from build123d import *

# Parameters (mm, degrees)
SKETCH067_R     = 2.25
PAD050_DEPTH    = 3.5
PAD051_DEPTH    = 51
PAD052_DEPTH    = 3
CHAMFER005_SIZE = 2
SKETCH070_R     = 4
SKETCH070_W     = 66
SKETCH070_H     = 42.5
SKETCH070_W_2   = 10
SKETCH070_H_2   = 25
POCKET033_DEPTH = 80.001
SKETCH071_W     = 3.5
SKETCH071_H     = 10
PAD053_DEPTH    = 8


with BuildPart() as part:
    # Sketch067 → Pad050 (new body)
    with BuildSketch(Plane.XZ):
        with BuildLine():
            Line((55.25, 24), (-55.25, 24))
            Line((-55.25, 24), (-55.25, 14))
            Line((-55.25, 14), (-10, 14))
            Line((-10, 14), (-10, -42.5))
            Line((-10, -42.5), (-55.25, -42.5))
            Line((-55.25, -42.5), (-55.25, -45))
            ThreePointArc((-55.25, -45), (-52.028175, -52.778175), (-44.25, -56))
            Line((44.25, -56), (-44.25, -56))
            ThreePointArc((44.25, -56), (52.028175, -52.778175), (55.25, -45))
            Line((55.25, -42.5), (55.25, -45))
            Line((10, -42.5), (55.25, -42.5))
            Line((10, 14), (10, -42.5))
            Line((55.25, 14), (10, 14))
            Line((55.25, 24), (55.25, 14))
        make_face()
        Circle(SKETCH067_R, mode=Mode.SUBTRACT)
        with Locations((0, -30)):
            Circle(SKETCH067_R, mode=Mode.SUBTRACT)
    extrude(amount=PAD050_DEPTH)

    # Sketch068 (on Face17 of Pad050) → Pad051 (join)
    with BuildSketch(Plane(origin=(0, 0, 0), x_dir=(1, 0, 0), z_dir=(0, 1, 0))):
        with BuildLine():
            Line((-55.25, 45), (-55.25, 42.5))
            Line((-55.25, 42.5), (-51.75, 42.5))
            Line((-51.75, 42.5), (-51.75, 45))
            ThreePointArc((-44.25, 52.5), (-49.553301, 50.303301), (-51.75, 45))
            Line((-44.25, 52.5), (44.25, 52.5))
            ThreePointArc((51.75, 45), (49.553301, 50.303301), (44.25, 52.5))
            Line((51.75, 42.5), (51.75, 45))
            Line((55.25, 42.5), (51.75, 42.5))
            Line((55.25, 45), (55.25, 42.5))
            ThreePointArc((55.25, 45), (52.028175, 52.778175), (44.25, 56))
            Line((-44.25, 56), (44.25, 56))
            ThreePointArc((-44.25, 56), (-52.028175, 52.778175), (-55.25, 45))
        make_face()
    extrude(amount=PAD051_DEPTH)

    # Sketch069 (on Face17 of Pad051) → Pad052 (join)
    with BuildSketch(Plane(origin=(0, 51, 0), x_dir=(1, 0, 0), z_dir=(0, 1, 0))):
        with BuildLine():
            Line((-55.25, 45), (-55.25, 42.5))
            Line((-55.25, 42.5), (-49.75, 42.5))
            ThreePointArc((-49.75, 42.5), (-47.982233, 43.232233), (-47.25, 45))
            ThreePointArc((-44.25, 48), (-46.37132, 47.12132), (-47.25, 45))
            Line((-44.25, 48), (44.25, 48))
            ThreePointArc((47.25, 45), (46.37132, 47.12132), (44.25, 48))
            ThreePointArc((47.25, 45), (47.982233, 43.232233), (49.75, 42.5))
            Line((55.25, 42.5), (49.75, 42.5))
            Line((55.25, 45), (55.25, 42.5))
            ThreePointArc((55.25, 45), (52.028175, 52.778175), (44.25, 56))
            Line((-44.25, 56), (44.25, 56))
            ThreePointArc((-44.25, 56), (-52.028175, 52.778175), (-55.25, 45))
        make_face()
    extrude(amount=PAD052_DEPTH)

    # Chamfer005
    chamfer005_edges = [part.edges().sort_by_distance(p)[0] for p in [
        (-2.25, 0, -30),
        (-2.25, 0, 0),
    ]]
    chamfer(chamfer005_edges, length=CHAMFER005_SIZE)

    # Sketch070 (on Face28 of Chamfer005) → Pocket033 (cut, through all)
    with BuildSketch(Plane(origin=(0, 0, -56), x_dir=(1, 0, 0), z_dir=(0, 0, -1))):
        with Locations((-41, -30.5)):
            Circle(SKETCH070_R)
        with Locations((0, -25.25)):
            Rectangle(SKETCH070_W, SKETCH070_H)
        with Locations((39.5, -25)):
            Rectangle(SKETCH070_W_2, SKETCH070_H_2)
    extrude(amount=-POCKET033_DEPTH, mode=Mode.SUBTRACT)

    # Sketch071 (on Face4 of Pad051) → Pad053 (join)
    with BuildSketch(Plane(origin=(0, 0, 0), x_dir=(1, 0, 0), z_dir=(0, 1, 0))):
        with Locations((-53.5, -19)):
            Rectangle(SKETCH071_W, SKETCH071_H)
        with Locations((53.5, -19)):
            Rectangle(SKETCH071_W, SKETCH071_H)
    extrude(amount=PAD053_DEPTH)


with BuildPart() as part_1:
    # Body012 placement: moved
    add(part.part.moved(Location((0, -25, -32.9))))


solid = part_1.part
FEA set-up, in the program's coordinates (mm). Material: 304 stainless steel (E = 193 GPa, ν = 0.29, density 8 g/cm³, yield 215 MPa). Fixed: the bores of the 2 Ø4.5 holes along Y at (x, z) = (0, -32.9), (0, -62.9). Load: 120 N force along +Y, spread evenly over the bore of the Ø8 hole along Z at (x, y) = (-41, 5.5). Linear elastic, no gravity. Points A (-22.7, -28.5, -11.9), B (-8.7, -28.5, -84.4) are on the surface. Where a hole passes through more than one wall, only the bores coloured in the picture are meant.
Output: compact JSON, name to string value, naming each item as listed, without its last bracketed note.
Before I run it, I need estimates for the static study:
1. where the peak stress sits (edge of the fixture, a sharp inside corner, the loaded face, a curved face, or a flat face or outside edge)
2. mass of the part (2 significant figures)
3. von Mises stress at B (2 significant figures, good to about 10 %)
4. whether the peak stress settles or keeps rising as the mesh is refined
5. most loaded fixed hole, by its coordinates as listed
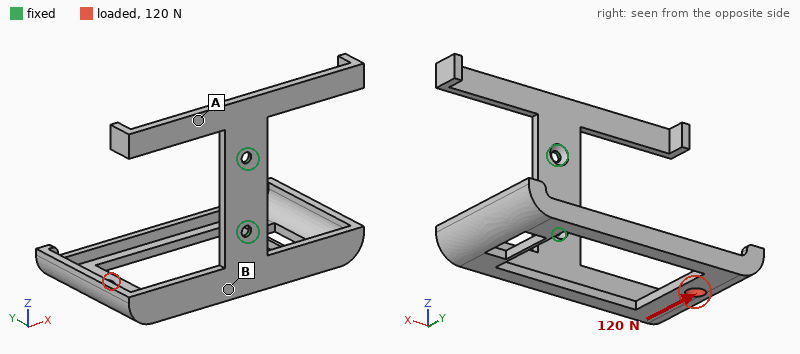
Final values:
{"where the peak stress sits": "edge of the fixture", "mass of the part": "220 g", "von Mises stress at B": "51 MPa", "whether the peak stress settles or keeps rising as the mesh is refined": "keeps rising", "most loaded fixed hole, by its coordinates as listed": "(0, -62.9)"}
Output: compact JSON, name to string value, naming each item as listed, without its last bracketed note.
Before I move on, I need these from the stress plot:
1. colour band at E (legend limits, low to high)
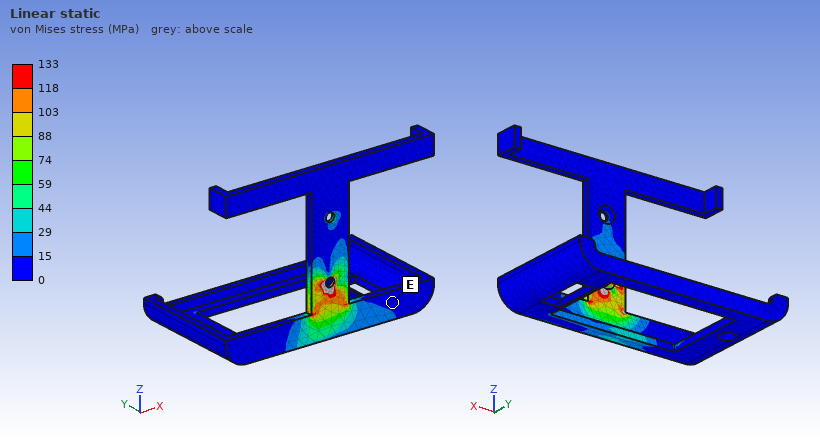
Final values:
{"colour band at E": "0 to 15 MPa"}
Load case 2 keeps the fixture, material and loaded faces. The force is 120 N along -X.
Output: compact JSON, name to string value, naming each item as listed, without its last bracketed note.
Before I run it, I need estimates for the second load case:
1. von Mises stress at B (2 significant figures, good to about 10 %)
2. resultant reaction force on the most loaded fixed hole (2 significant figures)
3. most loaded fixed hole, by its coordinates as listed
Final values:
{"von Mises stress at B": "33 MPa", "resultant reaction force on the most loaded fixed hole": "170 N", "most loaded fixed hole, by its coordinates as listed": "(0, -62.9)"}
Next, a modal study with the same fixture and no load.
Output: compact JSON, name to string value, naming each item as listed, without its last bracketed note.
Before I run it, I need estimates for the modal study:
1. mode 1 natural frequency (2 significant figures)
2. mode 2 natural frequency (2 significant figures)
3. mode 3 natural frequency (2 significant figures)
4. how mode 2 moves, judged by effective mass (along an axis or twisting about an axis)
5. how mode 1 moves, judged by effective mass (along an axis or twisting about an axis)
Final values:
{"mode 1 natural frequency": "220 Hz", "mode 2 natural frequency": "240 Hz", "mode 3 natural frequency": "570 Hz", "how mode 2 moves, judged by effective mass": "along Z", "how mode 1 moves, judged by effective mass": "along X"}
